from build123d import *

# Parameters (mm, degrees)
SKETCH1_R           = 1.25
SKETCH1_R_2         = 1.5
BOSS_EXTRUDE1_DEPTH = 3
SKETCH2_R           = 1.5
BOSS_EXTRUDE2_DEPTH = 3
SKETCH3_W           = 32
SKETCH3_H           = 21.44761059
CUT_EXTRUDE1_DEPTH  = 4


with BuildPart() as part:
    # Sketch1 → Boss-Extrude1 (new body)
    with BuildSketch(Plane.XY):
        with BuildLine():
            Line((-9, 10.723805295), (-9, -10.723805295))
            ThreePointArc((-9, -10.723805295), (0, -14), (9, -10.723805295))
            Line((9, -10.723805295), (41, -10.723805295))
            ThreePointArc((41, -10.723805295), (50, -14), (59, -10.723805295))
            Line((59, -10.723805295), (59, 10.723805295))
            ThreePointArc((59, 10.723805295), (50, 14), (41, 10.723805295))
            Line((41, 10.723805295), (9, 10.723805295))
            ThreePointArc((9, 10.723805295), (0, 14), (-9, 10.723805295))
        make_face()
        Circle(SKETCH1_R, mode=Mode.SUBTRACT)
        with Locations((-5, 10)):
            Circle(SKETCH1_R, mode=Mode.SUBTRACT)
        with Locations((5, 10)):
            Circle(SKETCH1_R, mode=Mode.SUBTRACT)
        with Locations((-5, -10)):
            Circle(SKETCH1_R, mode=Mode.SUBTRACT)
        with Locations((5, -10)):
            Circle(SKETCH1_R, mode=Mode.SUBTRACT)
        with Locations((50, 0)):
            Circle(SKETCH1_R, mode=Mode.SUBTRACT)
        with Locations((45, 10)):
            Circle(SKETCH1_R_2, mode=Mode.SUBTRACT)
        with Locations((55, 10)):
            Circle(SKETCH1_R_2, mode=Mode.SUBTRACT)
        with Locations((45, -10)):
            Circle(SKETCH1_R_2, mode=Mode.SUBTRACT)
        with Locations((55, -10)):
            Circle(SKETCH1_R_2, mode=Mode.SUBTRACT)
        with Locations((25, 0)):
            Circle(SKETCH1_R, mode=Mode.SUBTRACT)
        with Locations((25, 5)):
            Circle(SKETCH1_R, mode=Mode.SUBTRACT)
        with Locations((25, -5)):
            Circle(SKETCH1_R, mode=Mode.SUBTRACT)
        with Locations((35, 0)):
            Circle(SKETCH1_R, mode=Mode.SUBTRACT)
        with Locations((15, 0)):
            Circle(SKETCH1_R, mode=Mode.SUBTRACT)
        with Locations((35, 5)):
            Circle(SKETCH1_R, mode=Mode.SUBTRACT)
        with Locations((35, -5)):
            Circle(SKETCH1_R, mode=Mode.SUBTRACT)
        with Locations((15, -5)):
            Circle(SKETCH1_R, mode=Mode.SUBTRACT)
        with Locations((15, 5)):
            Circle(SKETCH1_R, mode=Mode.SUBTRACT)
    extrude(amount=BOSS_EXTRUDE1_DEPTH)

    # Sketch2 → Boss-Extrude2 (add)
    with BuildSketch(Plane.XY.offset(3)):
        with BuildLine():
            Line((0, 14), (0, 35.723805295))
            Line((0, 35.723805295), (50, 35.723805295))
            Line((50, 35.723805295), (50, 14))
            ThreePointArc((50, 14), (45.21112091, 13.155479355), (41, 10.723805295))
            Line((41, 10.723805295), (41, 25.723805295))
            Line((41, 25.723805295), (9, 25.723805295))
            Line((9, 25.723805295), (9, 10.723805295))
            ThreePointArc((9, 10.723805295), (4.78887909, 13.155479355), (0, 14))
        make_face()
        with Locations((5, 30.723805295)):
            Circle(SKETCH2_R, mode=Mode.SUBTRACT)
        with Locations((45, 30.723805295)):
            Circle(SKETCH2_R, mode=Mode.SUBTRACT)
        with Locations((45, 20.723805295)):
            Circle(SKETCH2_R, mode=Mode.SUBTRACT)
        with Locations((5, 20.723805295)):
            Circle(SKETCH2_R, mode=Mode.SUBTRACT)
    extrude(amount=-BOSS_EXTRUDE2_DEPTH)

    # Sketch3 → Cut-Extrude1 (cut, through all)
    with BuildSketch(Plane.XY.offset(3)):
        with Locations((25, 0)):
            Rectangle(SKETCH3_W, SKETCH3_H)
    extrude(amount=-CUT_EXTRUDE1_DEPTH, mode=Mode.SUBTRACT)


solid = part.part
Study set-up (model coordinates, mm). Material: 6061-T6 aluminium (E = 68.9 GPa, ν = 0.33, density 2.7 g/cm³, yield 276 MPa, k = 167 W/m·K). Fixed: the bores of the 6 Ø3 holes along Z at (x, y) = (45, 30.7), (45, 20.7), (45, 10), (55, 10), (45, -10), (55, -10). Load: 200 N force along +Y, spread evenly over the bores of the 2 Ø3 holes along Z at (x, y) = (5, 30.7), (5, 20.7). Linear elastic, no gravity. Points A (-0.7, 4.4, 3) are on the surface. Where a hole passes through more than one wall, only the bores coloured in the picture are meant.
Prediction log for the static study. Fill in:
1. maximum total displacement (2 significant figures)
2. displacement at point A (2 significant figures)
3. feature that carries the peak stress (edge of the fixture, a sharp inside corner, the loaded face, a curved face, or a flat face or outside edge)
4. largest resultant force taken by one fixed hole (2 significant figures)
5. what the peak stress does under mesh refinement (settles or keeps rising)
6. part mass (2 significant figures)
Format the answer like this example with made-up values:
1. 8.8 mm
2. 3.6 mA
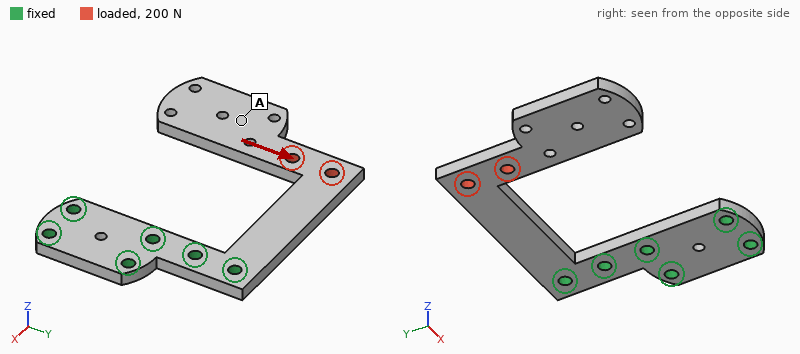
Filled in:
1. 0.58 mm
2. 0.42 mm
3. edge of the fixture
4. 650 N
5. keeps rising
6. 13 g
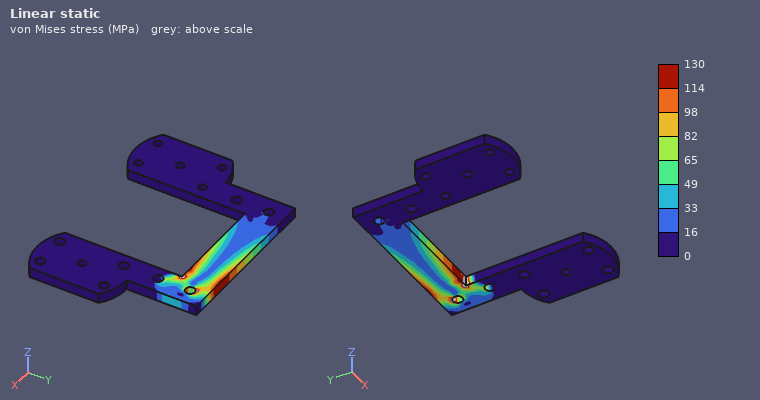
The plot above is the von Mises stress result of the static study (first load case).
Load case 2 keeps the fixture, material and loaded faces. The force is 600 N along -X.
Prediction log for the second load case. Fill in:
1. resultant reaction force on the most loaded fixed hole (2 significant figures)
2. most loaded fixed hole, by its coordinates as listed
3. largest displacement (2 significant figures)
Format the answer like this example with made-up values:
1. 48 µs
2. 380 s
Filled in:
1. 360 N
2. (45, 30.7)
3. 0.41 mm
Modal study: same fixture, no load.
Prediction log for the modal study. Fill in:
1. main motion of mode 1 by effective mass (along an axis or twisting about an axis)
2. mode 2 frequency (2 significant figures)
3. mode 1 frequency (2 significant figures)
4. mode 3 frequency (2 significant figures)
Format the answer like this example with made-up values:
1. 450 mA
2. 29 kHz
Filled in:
1. along Z
2. 1100 Hz
3. 380 Hz
4. 1300 Hz
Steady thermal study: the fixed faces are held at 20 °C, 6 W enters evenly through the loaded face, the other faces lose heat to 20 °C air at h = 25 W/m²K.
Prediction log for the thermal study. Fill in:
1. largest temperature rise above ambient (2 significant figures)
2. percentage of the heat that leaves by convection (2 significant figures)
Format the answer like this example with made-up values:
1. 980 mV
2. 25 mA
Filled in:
1. 36 K
2. 30 %
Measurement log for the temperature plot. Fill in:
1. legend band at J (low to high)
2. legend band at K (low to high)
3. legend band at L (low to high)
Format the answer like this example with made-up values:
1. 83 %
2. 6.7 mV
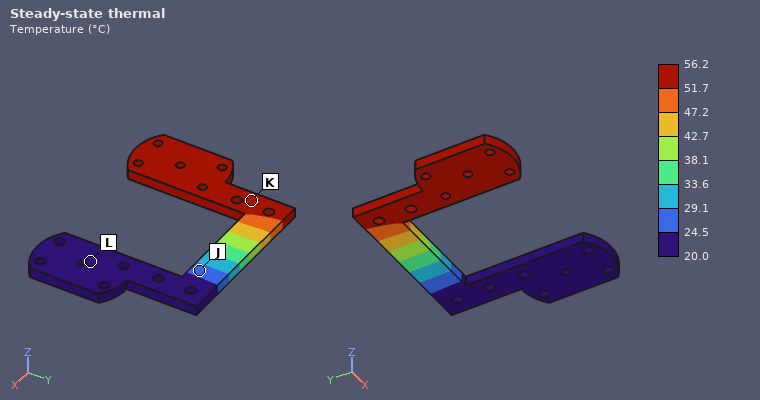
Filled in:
1. 24.5 to 29.1 °C
2. 51.7 to 56.2 °C
3. 20.0 to 24.5 °C
